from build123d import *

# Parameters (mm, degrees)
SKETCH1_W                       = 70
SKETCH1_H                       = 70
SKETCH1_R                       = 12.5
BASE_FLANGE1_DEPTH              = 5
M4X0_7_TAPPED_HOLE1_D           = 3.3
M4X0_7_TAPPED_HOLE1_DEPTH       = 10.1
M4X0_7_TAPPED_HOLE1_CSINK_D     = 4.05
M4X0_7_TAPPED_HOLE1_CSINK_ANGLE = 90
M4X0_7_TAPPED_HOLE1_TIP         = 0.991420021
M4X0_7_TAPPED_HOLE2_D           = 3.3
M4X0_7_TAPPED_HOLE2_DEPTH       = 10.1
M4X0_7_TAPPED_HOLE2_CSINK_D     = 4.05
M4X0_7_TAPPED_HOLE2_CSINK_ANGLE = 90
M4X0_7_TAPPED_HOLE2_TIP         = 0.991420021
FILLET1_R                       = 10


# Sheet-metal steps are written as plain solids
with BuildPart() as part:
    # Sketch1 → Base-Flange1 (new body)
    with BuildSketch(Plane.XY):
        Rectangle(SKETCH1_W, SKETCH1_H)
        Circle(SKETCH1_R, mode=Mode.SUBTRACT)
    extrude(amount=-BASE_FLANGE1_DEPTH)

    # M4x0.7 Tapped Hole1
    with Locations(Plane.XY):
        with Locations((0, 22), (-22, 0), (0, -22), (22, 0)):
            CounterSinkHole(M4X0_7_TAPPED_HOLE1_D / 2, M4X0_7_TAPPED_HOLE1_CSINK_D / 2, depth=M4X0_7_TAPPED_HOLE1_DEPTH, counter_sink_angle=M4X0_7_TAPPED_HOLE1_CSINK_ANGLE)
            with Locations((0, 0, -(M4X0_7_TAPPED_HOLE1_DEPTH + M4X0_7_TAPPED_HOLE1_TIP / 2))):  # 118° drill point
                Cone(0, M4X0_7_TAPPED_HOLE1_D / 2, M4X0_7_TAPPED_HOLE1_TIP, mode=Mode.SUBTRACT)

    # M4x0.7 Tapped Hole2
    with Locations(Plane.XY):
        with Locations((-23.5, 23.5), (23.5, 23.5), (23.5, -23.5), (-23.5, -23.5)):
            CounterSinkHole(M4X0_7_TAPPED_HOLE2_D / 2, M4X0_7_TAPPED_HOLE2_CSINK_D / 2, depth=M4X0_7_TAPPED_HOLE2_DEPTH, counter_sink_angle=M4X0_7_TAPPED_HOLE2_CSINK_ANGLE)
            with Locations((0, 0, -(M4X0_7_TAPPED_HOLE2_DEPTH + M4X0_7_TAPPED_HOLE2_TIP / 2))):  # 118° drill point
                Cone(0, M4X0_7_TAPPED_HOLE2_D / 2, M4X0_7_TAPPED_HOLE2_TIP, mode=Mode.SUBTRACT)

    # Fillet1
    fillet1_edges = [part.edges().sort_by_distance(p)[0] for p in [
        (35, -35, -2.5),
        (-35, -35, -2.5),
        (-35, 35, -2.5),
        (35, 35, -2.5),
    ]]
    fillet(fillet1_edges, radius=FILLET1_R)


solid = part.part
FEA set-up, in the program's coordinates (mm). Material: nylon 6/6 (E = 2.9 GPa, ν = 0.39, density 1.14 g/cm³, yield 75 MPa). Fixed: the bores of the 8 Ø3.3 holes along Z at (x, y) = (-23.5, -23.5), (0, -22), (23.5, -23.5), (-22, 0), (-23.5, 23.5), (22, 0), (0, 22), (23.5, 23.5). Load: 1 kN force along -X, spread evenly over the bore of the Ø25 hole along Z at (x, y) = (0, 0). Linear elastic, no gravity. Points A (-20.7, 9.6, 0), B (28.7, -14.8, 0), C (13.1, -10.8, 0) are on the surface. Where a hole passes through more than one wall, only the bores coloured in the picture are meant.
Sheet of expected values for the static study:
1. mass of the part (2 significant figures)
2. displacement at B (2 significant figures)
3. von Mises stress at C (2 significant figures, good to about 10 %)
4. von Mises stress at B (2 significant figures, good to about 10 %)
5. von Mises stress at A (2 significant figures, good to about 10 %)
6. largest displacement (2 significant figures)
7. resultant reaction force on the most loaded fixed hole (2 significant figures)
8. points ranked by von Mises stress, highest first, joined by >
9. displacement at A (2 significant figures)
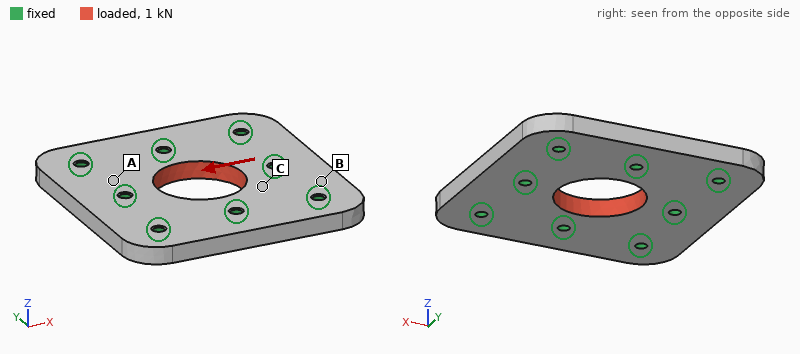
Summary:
24 g
5.2 µm
2.0 MPa
0.59 MPa
1.1 MPa
17 µm
230 N
C > A > B
7.8 µm
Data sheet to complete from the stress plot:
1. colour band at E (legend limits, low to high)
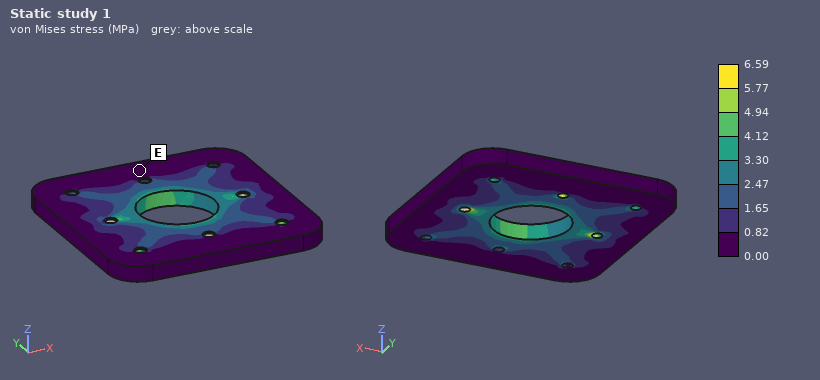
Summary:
0.00 to 0.82 MPa
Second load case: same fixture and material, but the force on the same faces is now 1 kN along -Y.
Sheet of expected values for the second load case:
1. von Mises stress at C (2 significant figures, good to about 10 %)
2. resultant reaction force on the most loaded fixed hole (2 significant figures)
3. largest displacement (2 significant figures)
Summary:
2.1 MPa
230 N
17 µm
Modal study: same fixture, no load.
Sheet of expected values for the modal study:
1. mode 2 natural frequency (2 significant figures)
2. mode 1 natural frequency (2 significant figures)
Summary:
6300 Hz
6100 Hz
